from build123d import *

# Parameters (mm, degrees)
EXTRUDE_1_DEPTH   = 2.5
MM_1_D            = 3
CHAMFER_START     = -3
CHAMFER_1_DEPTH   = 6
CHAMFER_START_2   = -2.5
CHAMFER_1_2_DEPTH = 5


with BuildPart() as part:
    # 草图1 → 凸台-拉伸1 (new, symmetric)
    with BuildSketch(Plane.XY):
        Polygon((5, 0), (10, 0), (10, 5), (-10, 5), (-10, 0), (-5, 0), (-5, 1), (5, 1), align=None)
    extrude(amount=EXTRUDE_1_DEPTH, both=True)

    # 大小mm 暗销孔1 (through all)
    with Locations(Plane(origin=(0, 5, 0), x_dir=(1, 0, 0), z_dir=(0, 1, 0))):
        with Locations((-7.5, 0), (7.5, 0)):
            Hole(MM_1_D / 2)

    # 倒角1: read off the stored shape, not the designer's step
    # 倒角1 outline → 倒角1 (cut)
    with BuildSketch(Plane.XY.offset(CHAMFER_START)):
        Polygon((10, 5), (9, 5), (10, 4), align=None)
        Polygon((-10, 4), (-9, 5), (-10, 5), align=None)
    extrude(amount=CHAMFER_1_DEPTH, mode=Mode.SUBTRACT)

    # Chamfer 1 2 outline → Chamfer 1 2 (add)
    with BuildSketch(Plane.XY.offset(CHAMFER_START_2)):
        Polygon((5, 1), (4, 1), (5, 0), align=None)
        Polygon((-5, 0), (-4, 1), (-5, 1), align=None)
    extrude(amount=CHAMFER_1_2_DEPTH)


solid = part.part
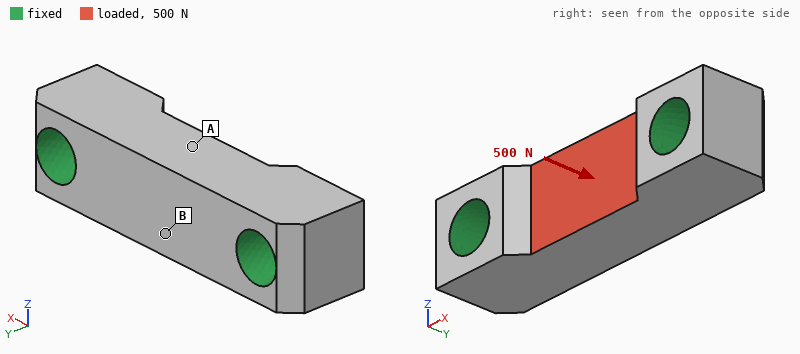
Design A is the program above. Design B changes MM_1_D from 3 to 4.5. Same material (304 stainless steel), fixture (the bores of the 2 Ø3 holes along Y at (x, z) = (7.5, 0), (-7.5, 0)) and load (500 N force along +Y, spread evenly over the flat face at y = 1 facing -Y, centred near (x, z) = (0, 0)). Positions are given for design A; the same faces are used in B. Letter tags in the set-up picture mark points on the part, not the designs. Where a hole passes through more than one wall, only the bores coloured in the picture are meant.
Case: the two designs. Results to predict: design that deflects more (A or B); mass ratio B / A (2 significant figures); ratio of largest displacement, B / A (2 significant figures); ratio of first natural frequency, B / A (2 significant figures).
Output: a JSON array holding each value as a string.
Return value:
["A", "0.77", "0.77", "1.2"]
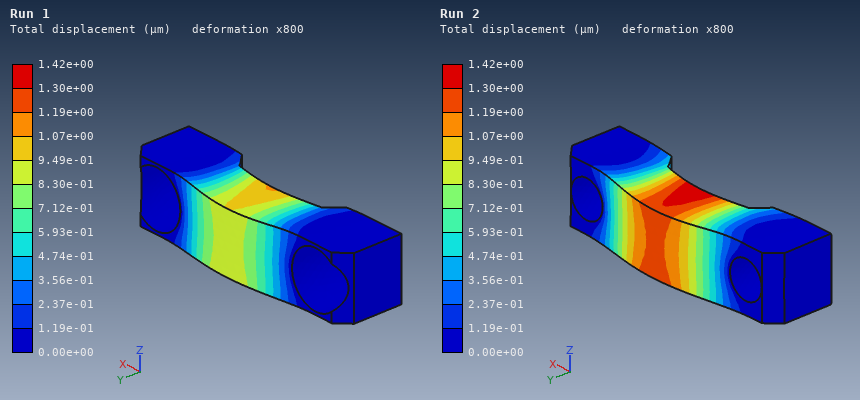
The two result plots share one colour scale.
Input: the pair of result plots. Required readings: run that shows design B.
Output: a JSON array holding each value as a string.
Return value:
["Run 1"]
